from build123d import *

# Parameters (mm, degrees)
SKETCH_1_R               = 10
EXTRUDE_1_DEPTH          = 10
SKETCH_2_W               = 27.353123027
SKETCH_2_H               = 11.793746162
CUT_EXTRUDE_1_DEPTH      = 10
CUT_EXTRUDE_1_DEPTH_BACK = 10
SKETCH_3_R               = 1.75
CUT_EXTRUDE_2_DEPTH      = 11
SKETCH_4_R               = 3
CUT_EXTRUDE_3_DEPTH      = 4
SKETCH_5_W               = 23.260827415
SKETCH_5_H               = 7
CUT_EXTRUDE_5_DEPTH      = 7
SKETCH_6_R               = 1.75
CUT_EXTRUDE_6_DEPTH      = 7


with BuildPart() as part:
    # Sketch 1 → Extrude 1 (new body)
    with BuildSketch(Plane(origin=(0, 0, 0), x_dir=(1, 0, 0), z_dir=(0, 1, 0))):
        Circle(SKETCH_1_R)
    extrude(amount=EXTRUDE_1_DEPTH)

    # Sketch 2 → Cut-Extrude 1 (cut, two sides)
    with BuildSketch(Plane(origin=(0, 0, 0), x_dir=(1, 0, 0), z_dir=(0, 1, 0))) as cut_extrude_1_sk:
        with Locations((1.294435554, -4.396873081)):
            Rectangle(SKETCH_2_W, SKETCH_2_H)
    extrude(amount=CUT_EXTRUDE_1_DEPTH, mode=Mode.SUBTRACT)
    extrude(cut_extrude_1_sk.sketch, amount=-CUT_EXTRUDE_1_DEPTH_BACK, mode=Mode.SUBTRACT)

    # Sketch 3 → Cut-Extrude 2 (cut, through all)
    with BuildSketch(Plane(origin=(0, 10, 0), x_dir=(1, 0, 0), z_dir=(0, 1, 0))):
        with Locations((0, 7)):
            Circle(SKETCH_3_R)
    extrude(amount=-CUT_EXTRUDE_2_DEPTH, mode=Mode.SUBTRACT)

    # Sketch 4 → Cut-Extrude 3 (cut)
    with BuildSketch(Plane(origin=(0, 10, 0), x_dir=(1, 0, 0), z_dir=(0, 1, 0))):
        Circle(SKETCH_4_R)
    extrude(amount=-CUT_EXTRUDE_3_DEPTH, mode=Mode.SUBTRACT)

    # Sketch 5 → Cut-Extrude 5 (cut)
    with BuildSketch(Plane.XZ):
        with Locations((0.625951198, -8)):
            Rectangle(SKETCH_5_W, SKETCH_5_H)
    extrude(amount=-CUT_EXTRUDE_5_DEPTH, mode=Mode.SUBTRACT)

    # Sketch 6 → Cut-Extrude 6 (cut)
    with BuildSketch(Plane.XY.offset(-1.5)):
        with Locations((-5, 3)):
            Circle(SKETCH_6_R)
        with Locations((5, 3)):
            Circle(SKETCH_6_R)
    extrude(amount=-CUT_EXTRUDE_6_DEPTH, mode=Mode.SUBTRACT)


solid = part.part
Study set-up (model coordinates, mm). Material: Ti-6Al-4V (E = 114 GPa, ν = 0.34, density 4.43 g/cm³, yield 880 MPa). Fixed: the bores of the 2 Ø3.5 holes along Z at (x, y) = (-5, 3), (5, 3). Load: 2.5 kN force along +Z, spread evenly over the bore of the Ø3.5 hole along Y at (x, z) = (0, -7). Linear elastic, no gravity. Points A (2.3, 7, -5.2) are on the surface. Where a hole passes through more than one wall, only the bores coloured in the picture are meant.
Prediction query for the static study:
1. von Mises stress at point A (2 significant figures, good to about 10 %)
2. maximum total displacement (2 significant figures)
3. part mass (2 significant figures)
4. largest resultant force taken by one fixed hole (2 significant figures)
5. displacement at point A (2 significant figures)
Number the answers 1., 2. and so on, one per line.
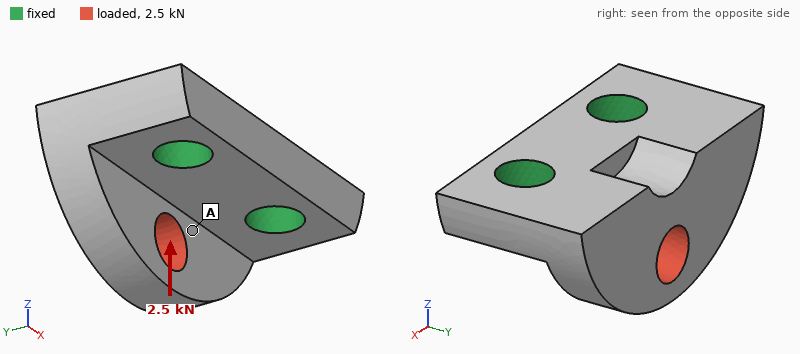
1. 110 MPa
2. 64 µm
3. 3.0 g
4. 1.3 kN
5. 22 µm
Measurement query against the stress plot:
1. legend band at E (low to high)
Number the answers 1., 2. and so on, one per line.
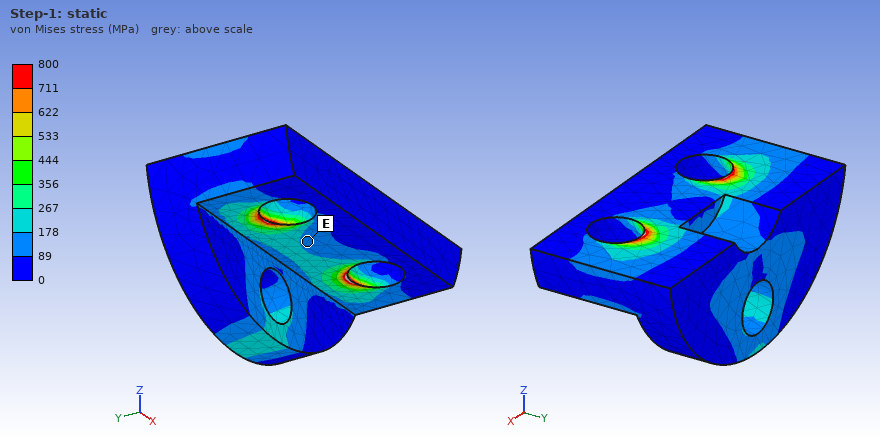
1. 89 to 178 MPa
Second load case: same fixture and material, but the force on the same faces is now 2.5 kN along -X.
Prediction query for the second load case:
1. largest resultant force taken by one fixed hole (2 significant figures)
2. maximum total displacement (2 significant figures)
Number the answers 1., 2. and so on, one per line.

1. 1.7 kN
2. 27 µm
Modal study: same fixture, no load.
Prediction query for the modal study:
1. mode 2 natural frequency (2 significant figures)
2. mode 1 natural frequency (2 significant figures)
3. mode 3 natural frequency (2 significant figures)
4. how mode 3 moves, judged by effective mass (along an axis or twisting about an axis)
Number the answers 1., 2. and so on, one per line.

1. 45 kHz
2. 30 kHz
3. 66 kHz
4. along X
